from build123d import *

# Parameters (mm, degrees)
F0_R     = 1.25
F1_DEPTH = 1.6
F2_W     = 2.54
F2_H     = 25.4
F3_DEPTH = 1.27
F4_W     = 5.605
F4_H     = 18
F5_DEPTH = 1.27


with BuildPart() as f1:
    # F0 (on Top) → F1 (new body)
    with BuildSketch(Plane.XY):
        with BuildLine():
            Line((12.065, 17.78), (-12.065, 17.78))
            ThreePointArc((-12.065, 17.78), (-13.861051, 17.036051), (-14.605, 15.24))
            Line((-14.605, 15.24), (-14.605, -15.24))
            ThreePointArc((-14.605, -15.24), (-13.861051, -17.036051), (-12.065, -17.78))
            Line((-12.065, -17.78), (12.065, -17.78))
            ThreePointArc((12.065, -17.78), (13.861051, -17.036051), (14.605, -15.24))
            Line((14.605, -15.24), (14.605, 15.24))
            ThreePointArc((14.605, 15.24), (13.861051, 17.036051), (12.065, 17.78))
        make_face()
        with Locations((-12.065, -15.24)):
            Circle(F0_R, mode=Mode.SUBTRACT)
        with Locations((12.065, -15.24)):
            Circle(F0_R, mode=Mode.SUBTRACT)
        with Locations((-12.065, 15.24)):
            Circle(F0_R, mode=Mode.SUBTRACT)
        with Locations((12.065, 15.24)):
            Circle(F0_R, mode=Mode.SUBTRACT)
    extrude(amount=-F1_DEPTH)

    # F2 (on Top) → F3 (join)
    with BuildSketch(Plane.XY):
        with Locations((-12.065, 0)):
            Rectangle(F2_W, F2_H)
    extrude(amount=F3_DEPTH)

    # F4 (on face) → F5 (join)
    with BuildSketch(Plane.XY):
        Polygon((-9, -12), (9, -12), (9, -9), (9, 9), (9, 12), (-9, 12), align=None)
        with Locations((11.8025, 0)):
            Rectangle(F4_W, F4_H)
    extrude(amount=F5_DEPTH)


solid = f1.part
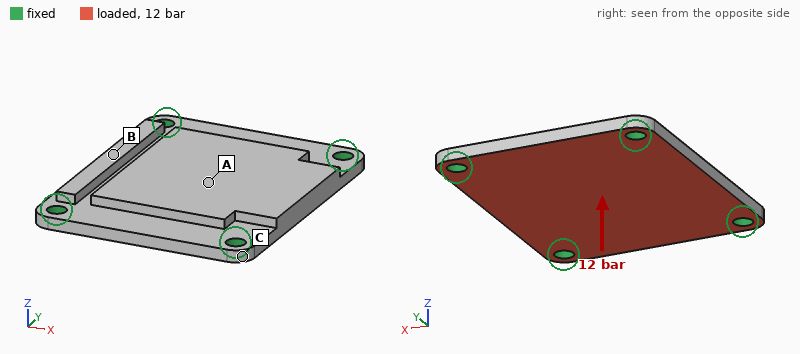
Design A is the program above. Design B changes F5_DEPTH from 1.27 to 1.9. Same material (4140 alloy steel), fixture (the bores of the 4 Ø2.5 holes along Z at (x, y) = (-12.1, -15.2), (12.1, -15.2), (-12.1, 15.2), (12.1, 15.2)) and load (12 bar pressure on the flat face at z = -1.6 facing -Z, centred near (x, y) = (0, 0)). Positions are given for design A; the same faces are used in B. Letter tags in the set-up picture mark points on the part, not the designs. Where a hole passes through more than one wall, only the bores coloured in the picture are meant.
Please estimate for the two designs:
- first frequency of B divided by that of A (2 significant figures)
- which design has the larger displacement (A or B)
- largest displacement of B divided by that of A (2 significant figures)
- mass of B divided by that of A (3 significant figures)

1.1
A
0.74
1.14
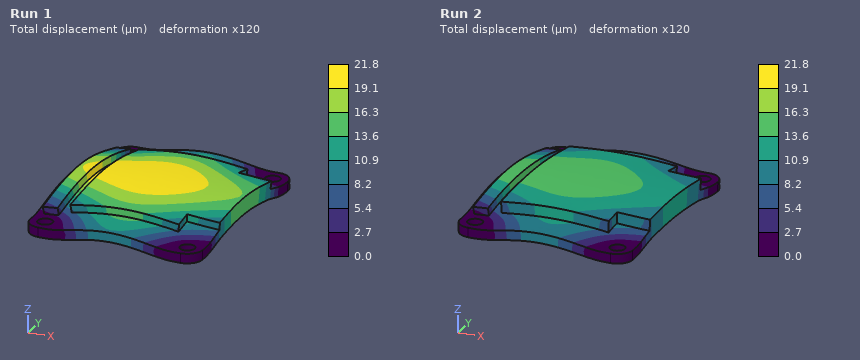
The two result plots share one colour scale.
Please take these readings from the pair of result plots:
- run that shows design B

Run 2
